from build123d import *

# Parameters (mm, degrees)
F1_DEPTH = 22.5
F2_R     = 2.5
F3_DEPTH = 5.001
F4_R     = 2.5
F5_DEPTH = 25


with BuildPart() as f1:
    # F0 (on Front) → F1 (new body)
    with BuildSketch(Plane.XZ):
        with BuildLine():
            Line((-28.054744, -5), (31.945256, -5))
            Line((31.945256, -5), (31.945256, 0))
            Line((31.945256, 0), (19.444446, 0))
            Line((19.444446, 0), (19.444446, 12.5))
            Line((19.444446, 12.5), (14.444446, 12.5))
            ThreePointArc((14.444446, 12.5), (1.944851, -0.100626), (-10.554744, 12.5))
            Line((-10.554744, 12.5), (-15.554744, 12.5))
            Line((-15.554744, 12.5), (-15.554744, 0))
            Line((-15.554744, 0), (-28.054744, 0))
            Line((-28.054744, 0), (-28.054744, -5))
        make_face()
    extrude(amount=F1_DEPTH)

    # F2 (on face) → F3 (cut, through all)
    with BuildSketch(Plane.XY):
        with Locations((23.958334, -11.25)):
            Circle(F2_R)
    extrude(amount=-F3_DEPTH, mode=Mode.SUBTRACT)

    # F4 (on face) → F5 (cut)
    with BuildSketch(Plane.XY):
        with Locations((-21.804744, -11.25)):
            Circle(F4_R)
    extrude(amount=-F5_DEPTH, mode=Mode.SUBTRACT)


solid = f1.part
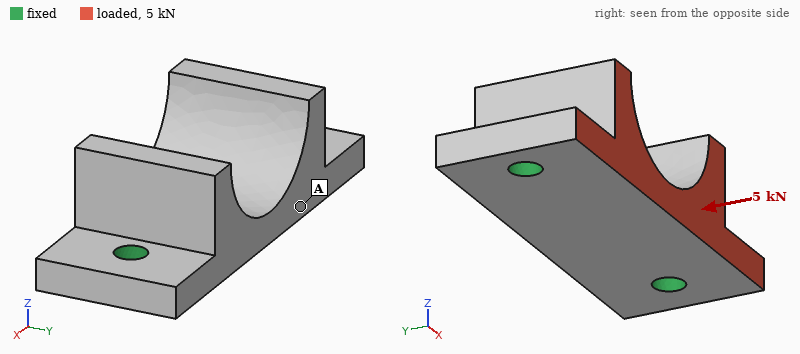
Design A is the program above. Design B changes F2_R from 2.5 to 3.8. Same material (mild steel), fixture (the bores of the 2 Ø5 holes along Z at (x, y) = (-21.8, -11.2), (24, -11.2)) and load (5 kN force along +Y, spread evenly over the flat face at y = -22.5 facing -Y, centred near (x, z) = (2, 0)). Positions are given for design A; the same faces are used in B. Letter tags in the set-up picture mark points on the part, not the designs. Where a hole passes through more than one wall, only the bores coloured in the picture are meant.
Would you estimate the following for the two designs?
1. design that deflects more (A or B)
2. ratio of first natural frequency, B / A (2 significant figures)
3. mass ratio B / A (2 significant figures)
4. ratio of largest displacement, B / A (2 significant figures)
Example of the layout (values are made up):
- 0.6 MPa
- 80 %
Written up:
- A
- 1.1
- 0.99
- 0.89
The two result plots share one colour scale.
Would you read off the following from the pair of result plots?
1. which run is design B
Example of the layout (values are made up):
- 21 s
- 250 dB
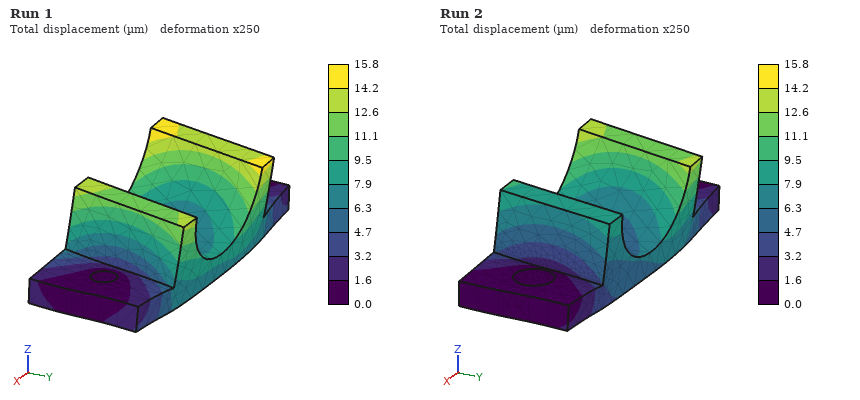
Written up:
- Run 2
